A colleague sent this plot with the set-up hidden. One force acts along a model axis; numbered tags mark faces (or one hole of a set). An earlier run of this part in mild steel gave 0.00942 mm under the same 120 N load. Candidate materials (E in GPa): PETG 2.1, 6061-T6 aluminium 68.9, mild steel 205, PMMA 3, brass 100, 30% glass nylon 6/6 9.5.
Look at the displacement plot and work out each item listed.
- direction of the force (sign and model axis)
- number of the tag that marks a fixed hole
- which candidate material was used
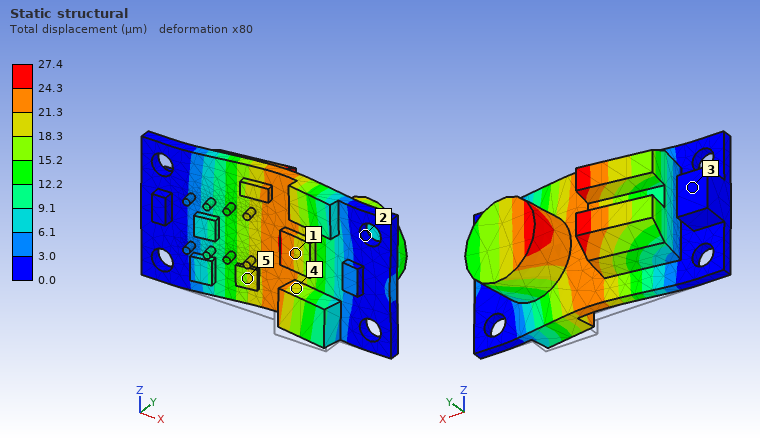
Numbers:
+Y
2
6061-T6 aluminium
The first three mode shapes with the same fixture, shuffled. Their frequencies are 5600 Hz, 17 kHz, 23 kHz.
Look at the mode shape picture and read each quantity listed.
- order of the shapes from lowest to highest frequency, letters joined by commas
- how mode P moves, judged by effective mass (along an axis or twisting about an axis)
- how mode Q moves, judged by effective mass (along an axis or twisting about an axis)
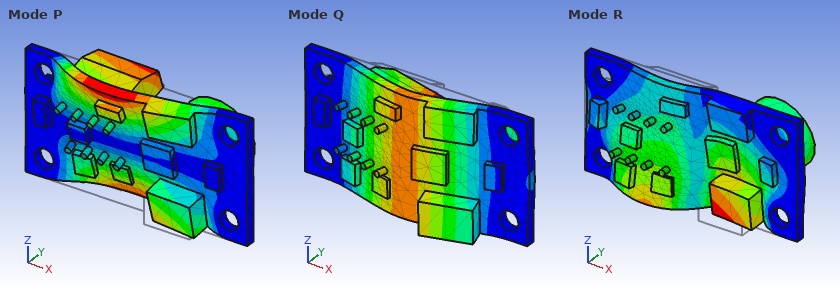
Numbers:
Q, P, R
along Z
along Y
